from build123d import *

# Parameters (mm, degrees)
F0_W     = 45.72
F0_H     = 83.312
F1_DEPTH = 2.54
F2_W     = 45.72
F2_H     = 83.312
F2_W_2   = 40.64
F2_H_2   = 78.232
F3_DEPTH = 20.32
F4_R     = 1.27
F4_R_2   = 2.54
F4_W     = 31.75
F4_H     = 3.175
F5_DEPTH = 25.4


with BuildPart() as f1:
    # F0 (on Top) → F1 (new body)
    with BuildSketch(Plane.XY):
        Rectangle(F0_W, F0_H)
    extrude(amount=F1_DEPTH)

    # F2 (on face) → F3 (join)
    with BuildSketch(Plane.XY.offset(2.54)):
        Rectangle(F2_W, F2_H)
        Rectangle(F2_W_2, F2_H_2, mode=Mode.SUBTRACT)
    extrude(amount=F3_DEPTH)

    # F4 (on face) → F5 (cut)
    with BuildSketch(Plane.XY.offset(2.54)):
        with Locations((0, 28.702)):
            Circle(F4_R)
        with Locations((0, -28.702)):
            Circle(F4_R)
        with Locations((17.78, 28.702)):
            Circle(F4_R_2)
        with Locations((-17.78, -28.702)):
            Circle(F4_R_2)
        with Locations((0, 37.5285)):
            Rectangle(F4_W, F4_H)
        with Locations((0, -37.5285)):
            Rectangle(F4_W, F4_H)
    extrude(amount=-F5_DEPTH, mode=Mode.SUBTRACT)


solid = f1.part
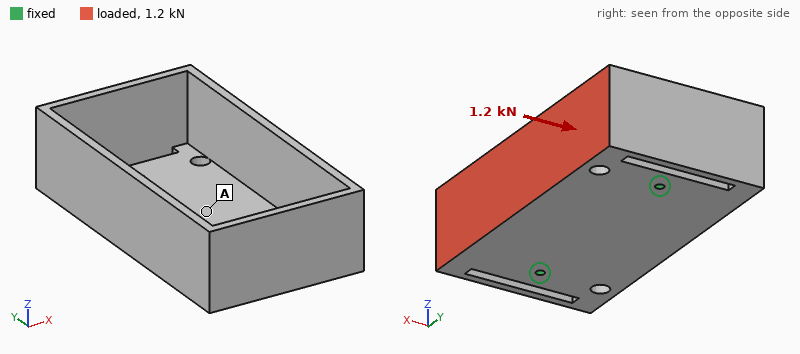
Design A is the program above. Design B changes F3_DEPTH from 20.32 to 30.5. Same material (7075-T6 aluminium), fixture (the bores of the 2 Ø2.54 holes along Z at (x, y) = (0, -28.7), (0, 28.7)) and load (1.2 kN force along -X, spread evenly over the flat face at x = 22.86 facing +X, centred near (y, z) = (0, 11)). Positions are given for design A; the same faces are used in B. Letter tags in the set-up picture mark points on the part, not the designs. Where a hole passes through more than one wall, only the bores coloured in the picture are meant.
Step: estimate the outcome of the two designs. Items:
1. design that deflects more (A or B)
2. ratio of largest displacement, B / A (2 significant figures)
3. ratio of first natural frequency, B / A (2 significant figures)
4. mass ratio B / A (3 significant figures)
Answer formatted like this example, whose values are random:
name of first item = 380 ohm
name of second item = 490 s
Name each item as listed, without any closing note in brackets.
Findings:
design that deflects more = B
ratio of largest displacement, B / A = 1.7
ratio of first natural frequency, B / A = 0.73
mass ratio B / A = 1.29
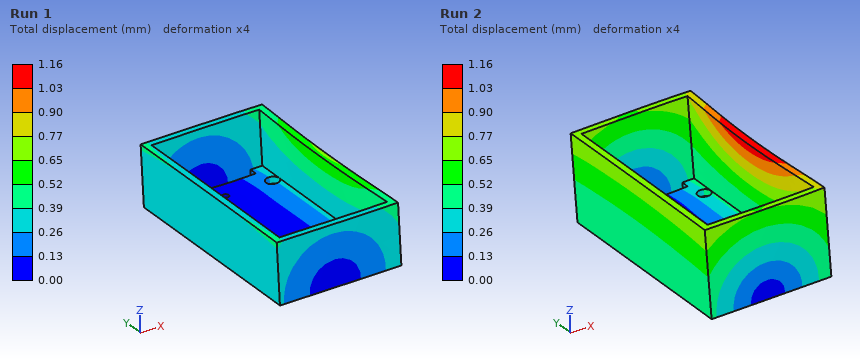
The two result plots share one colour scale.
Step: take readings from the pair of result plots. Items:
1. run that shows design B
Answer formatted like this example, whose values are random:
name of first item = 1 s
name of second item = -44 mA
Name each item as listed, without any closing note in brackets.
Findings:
run that shows design B = Run 2
